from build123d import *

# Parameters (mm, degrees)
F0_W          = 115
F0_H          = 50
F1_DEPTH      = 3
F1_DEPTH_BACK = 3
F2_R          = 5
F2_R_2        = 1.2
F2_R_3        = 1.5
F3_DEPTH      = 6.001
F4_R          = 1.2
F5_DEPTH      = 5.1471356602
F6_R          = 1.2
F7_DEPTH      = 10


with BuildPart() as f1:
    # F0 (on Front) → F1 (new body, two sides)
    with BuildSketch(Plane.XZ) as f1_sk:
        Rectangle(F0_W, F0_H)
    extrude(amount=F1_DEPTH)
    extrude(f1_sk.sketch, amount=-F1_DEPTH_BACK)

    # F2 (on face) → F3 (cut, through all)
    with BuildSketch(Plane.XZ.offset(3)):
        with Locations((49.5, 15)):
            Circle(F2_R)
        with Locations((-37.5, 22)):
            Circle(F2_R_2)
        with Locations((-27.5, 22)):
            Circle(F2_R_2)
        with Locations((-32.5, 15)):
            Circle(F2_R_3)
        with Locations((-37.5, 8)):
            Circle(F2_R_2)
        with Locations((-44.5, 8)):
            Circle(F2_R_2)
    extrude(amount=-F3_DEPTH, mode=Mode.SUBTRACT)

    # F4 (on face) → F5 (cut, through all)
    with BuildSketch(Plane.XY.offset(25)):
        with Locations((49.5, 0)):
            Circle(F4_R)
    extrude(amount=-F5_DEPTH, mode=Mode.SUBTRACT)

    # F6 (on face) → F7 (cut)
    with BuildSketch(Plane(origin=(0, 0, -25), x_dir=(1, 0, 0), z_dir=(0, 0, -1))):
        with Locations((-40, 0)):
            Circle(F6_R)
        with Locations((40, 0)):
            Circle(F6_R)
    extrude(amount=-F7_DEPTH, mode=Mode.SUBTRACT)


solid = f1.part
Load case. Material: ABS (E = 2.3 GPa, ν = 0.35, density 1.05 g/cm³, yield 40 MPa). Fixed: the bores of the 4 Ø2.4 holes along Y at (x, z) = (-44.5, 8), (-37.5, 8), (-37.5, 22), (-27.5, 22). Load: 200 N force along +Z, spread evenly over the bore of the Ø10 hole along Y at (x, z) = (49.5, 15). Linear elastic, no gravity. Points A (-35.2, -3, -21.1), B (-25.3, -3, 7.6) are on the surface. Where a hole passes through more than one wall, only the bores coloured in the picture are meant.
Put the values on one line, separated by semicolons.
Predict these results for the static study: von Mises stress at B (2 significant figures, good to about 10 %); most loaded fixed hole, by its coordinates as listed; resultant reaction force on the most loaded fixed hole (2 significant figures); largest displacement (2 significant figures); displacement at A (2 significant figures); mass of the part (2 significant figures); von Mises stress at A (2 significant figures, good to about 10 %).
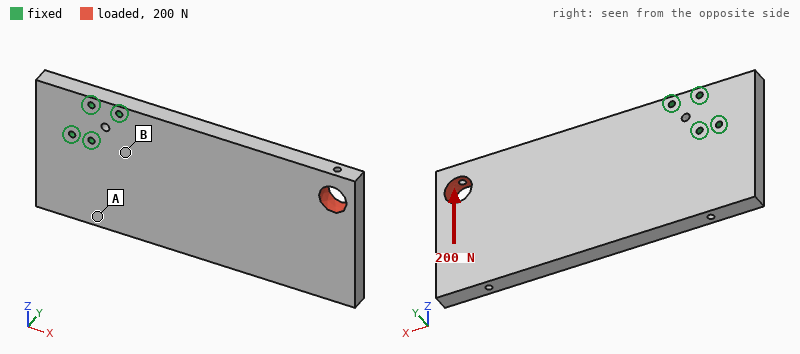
4.9 MPa; (-27.5, 22); 650 N; 0.81 mm; 0.19 mm; 35 g; 2.1 MPa
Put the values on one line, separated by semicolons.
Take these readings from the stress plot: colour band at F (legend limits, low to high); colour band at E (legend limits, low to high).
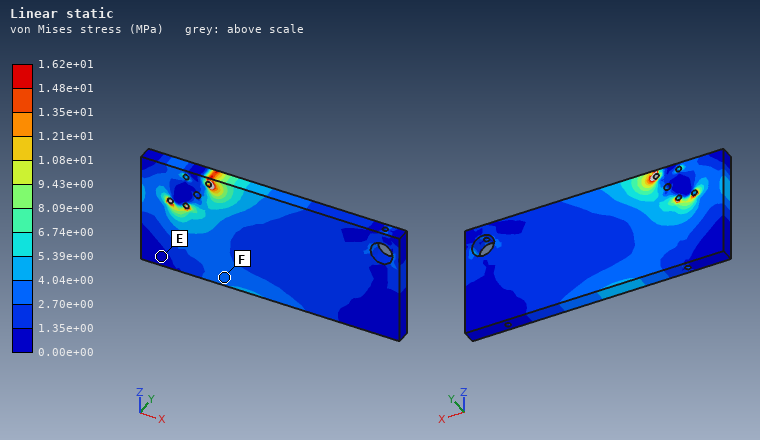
2.70e+00 to 4.04e+00 MPa; 0.00e+00 to 1.35e+00 MPa
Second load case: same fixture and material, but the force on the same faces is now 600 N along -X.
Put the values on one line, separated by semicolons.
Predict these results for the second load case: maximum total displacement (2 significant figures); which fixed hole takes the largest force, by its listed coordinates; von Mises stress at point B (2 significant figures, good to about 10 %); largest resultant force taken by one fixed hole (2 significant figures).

0.28 mm; (-27.5, 22); 2.9 MPa; 280 N
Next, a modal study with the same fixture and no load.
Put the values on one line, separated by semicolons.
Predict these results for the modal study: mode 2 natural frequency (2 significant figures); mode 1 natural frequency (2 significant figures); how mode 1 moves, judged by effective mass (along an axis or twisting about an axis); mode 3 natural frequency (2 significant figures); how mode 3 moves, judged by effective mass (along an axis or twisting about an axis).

570 Hz; 160 Hz; along Y; 800 Hz; along Z
